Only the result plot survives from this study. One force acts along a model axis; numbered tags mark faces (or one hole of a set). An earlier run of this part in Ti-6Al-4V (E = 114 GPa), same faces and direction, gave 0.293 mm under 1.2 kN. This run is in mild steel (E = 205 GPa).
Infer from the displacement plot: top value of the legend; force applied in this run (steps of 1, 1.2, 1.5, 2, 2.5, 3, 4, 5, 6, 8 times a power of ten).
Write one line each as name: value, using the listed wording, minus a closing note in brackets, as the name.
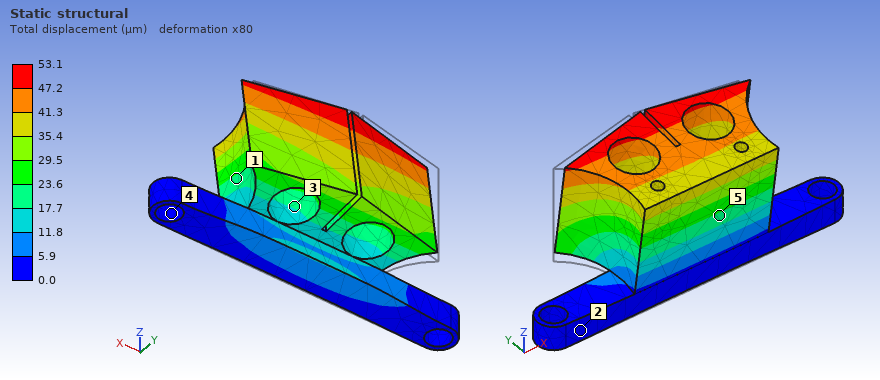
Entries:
top value of the legend: 53.1 µm
force applied in this run: 400 N
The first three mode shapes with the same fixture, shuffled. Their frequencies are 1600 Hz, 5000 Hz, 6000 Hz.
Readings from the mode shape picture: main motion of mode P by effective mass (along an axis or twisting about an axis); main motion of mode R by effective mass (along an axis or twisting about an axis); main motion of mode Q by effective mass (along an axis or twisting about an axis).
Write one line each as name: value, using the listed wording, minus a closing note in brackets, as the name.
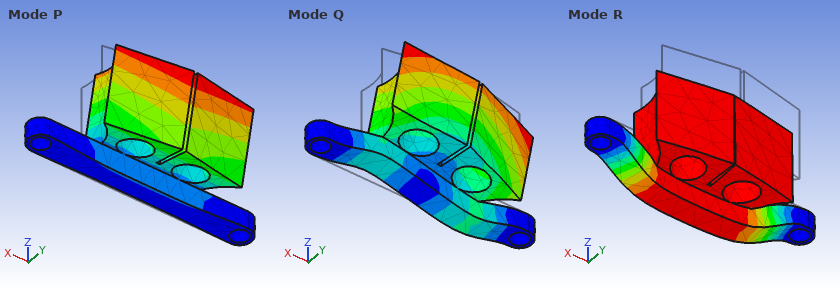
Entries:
main motion of mode P by effective mass: along Y
main motion of mode R by effective mass: along Z
main motion of mode Q by effective mass: along X
